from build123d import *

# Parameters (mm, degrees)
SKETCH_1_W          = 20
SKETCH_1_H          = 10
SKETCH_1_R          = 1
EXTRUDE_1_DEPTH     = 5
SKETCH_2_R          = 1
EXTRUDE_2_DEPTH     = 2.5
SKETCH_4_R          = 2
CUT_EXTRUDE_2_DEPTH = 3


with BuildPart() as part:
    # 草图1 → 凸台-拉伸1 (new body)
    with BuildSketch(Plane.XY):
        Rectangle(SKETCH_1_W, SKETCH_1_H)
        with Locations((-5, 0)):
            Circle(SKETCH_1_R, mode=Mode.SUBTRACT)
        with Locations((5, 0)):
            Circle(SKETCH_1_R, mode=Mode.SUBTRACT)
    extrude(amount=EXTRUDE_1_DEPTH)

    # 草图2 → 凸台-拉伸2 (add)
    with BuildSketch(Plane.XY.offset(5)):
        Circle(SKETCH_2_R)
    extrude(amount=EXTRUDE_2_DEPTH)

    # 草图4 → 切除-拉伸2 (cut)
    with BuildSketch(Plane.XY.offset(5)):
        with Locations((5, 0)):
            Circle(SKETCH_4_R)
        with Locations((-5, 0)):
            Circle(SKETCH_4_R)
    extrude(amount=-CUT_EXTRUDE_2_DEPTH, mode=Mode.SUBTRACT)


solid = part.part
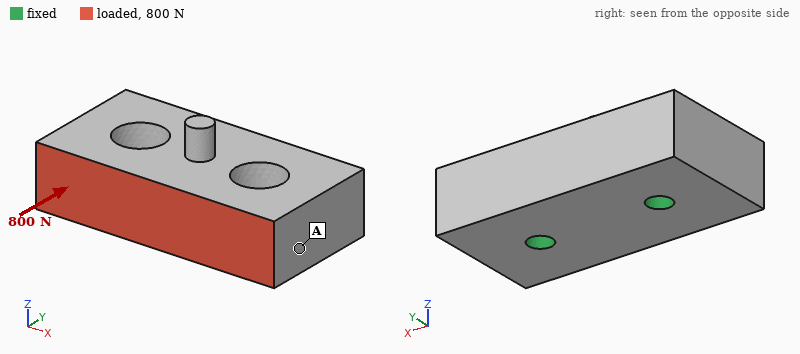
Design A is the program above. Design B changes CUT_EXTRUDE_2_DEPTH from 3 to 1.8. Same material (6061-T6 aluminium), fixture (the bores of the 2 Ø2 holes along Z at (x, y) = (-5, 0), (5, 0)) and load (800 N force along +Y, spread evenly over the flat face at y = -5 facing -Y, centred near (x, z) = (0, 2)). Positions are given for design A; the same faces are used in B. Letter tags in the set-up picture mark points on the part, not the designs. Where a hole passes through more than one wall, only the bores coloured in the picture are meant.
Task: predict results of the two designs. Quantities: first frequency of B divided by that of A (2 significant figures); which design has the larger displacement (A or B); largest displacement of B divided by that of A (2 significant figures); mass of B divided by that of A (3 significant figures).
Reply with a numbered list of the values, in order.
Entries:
1. 1.7
2. A
3. 0.32
4. 1.02
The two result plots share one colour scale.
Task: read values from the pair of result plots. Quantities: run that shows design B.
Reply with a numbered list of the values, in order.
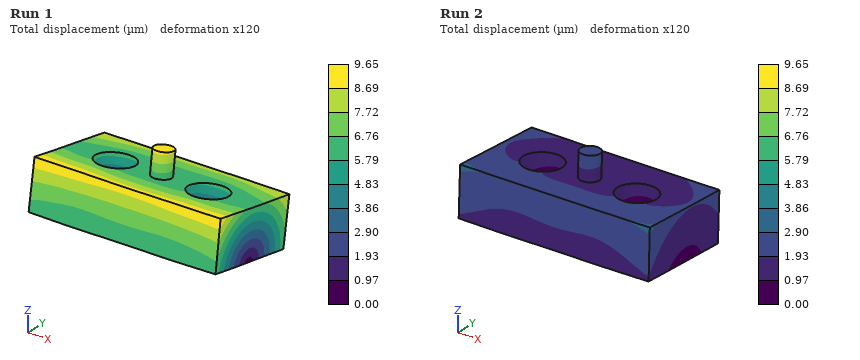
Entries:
1. Run 2
